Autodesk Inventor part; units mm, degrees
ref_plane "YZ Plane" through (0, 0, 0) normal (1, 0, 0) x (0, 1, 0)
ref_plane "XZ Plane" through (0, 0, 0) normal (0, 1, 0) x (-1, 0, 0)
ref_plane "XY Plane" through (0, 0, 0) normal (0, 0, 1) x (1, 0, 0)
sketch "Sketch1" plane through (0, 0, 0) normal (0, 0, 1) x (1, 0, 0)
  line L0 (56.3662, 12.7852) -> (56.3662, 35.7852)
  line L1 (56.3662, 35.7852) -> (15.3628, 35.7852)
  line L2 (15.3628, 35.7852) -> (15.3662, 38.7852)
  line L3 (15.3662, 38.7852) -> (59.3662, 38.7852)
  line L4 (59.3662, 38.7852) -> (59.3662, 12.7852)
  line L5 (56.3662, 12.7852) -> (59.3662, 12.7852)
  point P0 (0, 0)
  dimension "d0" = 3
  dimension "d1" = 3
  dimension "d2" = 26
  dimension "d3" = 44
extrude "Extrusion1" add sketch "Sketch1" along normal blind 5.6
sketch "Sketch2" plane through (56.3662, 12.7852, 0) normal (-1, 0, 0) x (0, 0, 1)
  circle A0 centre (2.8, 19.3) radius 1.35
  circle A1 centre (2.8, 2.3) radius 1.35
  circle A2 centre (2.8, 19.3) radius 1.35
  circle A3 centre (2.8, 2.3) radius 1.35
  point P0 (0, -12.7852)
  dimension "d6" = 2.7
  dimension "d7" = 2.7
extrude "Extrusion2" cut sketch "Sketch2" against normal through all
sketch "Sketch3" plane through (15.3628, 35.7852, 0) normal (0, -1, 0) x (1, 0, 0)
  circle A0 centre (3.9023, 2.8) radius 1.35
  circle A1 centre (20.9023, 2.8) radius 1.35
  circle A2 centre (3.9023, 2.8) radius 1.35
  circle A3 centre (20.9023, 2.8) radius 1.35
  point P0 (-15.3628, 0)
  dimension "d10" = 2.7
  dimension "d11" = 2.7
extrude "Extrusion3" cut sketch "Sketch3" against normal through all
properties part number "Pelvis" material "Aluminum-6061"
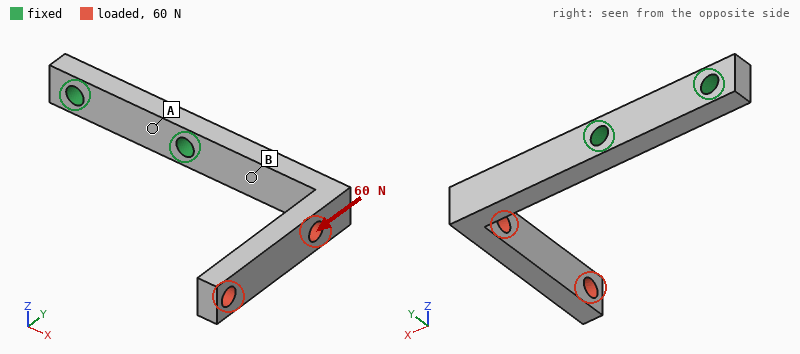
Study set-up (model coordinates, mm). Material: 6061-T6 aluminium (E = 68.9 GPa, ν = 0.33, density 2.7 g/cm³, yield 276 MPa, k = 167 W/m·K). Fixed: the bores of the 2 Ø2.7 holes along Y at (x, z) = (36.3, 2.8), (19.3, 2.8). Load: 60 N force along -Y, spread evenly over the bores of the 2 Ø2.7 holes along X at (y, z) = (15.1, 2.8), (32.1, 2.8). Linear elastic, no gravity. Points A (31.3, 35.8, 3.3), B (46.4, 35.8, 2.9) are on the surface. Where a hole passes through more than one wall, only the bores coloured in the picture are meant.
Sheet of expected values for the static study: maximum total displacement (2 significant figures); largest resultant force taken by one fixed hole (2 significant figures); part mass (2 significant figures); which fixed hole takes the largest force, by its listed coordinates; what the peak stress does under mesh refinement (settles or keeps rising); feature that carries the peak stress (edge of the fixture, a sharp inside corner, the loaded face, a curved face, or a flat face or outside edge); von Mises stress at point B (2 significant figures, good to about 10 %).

0.43 mm
62 N
2.9 g
(36.3, 2.8)
keeps rising
edge of the fixture
82 MPa
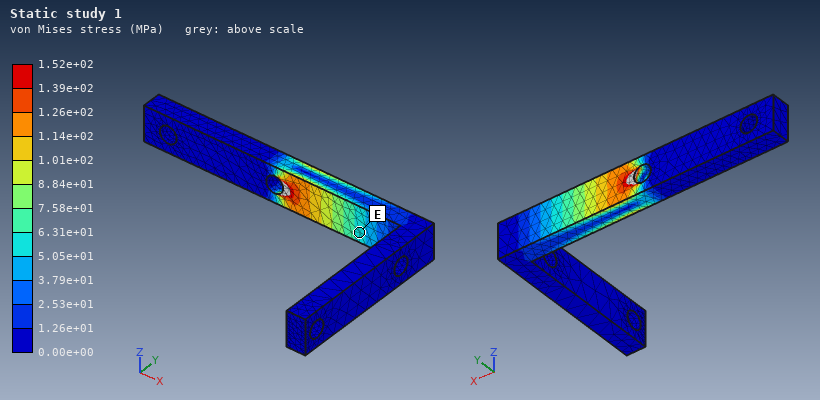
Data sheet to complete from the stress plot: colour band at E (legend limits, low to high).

5.05e+01 to 6.31e+01 MPa
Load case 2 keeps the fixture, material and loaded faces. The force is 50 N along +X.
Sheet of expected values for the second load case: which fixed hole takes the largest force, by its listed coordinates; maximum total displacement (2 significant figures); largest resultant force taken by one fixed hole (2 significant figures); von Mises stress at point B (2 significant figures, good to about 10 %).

(36.3, 2.8)
0.58 mm
49 N
84 MPa
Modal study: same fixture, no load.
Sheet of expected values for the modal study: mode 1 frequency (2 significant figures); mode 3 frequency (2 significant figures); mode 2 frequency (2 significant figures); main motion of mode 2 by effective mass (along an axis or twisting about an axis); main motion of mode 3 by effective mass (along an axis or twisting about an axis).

1700 Hz
4400 Hz
2100 Hz
along Z
along Y
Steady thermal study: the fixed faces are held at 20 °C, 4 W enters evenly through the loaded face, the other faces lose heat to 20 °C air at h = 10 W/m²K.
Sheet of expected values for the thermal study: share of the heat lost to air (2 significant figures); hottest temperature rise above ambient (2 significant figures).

5.4 %
49 K
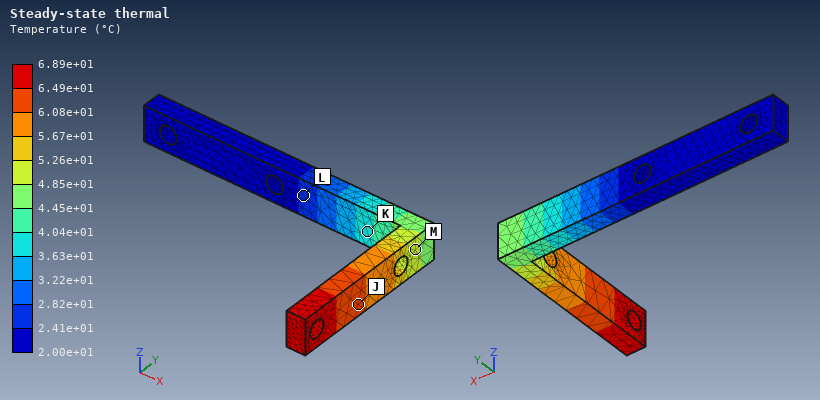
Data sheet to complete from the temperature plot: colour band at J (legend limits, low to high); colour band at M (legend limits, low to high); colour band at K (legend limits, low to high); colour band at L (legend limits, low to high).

6.08e+01 to 6.49e+01 °C
4.85e+01 to 5.26e+01 °C
3.63e+01 to 4.04e+01 °C
2.41e+01 to 2.82e+01 °C
